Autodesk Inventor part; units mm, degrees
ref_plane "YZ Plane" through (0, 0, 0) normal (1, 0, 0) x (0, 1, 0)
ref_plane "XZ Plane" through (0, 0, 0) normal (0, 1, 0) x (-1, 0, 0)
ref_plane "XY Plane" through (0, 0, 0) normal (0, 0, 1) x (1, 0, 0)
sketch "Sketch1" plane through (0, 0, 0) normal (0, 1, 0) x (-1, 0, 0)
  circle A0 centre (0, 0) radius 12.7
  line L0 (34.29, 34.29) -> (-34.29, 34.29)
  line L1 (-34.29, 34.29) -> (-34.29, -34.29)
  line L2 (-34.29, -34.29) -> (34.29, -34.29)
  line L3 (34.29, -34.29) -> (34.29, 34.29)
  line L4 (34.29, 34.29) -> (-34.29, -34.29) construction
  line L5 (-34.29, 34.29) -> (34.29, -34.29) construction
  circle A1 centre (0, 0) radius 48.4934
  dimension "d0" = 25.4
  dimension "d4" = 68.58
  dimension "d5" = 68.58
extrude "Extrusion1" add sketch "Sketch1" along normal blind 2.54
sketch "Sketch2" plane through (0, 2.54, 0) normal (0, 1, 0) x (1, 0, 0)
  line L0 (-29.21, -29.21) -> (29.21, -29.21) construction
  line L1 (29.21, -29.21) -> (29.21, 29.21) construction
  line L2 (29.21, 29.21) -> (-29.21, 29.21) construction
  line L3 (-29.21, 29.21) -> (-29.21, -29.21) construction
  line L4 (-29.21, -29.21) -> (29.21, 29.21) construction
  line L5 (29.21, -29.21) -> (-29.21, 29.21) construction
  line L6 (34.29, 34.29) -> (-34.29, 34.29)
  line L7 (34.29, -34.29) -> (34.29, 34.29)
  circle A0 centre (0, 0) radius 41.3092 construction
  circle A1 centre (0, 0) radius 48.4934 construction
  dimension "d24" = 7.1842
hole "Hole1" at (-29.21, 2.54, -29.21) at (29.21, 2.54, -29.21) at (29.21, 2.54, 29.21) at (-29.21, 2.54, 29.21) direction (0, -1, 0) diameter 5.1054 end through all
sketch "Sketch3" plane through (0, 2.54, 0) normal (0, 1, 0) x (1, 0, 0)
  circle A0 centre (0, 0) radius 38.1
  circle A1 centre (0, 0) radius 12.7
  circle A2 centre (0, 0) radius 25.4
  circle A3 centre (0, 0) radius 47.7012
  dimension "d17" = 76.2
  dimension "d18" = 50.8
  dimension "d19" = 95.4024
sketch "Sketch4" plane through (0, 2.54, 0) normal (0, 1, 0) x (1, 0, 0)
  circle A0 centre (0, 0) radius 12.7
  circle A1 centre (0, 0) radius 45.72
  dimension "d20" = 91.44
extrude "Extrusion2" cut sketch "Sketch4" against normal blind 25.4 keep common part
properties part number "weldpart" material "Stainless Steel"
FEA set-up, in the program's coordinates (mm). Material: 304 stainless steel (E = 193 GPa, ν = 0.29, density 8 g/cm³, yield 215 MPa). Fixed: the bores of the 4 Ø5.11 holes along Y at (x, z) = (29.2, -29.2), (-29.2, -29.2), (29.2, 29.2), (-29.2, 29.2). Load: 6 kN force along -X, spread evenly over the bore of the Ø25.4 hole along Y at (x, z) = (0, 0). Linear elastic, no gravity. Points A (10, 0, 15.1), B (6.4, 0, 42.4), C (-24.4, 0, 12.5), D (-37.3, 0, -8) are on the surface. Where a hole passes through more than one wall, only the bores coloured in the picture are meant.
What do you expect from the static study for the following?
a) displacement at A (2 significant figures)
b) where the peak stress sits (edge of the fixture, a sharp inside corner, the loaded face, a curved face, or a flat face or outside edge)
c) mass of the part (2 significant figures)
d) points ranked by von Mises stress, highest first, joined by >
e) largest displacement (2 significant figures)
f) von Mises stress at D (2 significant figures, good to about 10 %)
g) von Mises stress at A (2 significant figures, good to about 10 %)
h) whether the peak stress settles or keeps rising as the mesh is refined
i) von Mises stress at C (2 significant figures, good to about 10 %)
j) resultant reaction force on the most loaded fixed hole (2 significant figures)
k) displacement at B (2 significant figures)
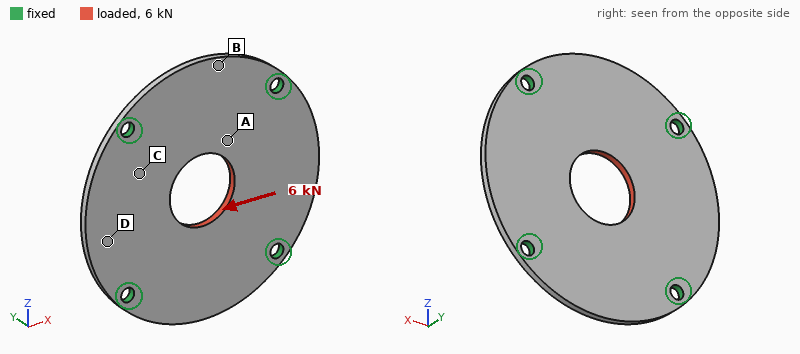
4.7 µm
edge of the fixture
120 g
A > C > D > B
7.1 µm
15 MPa
30 MPa
keeps rising
22 MPa
1.5 kN
1.4 µm
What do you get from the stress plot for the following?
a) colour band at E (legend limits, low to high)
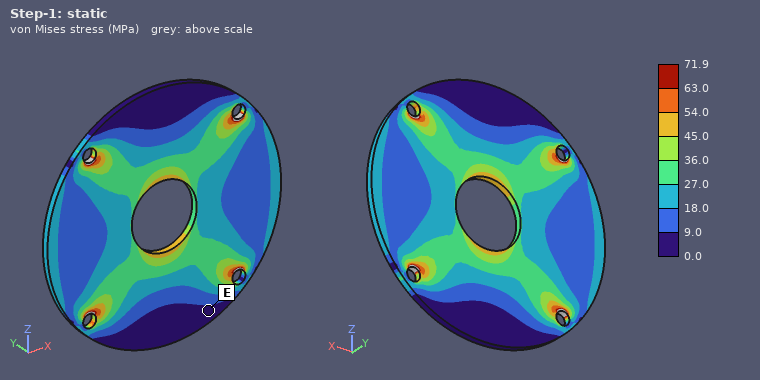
0.0 to 9.0 MPa
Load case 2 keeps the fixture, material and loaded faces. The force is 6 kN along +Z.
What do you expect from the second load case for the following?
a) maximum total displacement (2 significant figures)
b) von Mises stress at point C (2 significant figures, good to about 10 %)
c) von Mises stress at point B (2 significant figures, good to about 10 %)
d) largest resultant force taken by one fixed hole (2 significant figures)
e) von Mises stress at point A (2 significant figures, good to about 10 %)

7.1 µm
24 MPa
19 MPa
1.5 kN
26 MPa
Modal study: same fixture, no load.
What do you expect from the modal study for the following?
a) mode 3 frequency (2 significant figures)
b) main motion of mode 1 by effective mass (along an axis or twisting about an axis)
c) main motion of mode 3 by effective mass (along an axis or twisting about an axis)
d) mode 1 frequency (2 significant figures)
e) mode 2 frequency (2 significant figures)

3500 Hz
along Y
twisting about X
3000 Hz
3300 Hz
